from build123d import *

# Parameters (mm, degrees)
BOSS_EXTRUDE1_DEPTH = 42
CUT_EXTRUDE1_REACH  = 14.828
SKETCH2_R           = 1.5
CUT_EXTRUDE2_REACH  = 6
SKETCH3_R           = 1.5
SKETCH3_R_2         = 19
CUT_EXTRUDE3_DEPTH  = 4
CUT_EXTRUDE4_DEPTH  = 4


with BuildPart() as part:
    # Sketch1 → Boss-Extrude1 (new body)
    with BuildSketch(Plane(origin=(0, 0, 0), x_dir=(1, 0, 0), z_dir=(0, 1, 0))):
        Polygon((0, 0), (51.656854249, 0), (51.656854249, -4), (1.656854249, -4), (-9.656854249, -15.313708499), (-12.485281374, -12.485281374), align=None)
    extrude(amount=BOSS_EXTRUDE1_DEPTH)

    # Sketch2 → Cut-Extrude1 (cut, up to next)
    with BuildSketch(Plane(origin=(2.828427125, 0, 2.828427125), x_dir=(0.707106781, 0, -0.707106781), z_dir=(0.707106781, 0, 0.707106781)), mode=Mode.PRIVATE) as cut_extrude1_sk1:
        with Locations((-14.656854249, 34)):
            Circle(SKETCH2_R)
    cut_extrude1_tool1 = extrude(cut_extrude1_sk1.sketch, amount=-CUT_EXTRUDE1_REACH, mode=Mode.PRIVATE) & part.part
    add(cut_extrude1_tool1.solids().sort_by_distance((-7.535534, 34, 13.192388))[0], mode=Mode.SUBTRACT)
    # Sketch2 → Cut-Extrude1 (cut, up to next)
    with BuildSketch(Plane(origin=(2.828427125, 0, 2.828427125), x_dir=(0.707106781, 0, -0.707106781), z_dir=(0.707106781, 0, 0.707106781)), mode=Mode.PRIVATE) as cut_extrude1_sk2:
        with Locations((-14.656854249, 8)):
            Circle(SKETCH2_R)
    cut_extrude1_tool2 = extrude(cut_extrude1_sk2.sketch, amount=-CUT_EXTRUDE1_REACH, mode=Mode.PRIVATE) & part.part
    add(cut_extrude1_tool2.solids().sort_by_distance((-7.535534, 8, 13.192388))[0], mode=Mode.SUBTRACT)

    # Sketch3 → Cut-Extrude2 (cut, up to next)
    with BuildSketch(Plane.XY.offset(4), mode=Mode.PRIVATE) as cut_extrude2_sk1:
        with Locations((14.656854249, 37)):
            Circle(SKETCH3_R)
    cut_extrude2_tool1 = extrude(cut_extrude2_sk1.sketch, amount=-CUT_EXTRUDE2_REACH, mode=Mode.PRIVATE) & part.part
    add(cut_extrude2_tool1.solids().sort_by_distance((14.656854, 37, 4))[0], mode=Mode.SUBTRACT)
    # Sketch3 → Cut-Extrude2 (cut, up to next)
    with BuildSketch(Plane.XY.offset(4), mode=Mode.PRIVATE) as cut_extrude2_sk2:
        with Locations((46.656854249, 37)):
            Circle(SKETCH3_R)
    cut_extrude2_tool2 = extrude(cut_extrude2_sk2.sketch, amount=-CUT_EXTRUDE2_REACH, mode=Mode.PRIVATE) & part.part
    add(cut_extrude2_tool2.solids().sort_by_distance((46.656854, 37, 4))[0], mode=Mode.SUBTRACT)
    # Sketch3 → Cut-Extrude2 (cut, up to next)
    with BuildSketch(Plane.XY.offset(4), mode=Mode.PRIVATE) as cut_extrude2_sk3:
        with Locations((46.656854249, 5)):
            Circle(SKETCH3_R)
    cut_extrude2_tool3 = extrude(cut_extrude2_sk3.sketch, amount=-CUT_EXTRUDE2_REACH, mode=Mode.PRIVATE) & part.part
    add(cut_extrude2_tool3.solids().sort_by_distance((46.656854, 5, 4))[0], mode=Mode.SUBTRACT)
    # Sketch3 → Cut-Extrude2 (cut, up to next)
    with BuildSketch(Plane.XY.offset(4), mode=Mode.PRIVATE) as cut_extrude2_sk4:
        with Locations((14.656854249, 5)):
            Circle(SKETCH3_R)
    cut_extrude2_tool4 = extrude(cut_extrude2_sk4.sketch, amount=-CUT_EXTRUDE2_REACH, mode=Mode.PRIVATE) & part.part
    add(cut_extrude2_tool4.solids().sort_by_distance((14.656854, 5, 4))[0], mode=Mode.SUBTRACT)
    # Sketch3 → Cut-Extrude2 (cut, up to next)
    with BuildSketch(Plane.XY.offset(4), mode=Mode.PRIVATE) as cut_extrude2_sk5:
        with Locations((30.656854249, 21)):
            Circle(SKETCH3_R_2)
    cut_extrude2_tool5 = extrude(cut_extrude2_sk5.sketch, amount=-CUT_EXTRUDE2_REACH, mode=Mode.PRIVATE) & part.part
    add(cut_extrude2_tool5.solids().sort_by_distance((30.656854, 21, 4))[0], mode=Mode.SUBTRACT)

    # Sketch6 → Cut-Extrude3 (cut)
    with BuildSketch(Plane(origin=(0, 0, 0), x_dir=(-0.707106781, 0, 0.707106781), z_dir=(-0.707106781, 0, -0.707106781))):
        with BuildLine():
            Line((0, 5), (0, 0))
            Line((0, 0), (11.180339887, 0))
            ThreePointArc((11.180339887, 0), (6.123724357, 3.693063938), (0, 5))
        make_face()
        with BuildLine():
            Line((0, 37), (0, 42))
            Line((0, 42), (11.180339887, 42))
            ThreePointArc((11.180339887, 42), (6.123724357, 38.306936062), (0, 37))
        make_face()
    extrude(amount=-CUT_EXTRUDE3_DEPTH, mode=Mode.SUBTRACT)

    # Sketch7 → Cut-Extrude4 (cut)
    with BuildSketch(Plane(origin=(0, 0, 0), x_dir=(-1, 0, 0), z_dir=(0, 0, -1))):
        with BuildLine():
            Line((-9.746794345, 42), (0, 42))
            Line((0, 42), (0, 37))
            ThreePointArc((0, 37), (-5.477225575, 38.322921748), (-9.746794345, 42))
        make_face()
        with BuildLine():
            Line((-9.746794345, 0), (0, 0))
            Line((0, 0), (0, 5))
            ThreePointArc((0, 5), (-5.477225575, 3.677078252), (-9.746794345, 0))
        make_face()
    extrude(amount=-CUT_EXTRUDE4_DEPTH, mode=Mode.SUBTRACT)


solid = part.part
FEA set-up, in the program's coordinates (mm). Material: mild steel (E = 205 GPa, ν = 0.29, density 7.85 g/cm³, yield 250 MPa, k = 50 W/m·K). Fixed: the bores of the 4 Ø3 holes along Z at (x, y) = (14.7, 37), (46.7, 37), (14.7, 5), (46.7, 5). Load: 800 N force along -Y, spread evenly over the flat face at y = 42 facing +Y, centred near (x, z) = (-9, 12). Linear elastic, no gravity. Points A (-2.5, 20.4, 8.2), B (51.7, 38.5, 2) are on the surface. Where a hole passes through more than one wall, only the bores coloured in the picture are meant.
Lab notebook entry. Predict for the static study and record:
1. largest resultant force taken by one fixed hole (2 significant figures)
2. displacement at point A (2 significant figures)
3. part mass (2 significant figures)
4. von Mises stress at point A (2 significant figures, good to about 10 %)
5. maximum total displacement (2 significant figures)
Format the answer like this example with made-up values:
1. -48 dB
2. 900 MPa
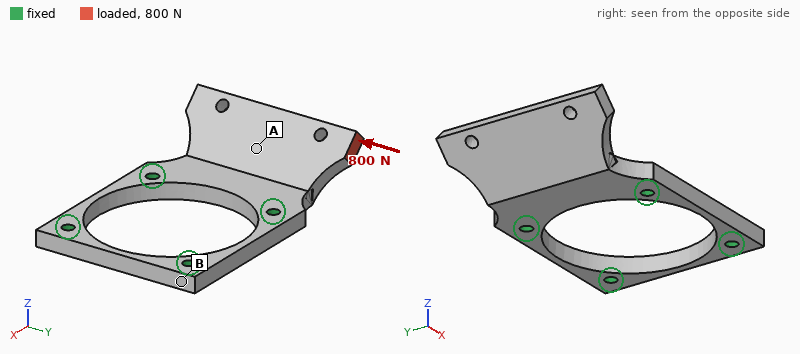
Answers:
1. 720 N
2. 6.7 µm
3. 48 g
4. 27 MPa
5. 26 µm
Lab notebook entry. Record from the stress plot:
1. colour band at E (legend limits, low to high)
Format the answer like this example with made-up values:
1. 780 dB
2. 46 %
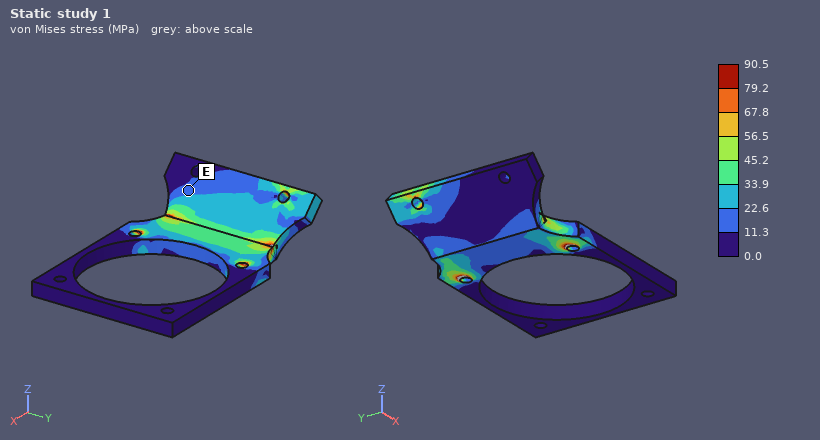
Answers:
1. 11.3 to 22.6 MPa
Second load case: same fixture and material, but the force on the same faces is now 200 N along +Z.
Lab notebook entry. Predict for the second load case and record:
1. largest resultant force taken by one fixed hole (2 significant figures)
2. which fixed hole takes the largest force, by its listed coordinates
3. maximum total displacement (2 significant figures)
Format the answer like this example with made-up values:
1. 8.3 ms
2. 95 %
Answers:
1. 230 N
2. (14.7, 37)
3. 77 µm
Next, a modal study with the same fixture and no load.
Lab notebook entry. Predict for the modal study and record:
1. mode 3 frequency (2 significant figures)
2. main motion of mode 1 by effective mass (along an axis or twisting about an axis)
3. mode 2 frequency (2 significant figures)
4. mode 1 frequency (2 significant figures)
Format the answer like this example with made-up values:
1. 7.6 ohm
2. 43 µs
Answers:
1. 13 kHz
2. along Z
3. 6600 Hz
4. 2900 Hz
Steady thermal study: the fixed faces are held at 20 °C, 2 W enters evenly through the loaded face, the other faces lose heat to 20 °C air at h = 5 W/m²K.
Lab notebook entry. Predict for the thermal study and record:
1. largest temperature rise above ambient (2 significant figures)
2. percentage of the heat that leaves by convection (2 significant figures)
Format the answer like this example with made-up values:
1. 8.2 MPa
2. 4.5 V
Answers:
1. 23 K
2. 4.4 %
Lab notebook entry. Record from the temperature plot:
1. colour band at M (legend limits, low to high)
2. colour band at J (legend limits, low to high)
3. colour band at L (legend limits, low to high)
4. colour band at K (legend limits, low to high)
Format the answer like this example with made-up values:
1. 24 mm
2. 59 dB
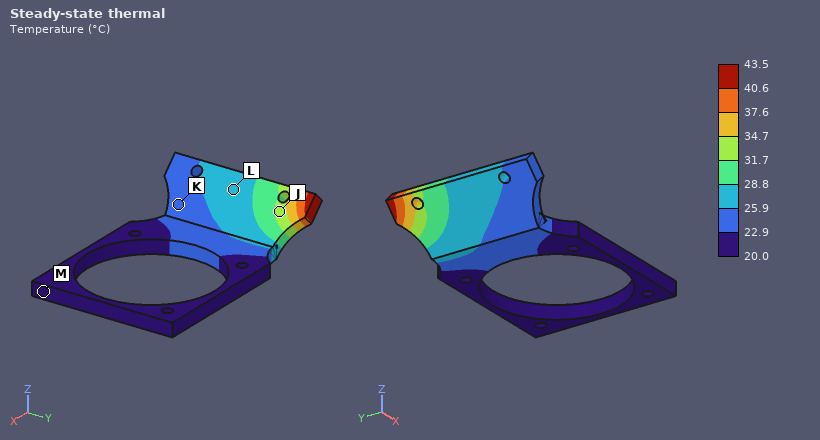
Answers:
1. 20.0 to 22.9 °C
2. 31.7 to 34.7 °C
3. 25.9 to 28.8 °C
4. 22.9 to 25.9 °C
